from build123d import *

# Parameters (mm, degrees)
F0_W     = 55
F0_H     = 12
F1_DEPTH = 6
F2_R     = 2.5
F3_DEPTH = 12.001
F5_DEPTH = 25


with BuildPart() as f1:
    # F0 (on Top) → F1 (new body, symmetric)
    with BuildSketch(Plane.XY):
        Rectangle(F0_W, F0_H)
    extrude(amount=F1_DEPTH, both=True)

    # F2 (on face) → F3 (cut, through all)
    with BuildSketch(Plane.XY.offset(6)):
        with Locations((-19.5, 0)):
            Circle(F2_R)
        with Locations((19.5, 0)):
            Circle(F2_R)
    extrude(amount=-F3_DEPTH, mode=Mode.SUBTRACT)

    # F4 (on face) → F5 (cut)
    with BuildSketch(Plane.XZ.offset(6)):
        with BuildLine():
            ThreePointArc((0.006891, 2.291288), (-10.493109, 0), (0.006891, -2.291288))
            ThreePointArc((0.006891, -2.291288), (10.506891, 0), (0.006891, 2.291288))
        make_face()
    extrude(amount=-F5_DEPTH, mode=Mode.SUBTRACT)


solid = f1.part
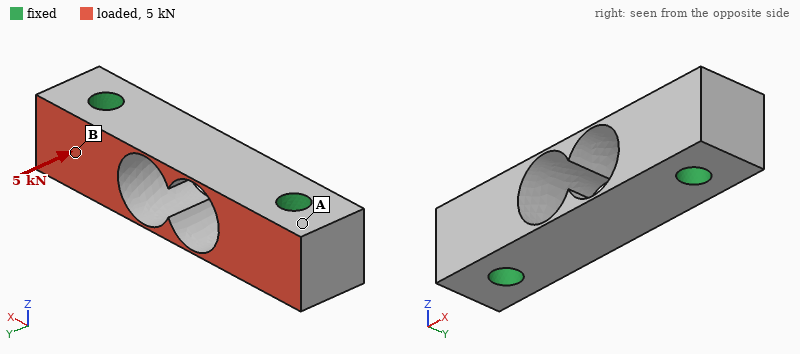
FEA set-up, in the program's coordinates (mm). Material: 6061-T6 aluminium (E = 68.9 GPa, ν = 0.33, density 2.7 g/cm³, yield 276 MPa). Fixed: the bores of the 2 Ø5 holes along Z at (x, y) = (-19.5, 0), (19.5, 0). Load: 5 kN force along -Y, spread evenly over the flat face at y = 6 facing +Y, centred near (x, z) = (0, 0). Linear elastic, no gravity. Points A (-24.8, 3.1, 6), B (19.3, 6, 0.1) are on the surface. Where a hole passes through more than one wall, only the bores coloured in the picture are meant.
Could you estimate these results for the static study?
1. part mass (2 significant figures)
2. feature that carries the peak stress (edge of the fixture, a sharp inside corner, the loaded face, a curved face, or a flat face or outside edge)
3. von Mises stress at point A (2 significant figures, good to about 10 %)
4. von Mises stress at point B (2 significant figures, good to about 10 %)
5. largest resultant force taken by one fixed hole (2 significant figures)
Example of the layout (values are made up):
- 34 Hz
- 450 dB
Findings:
- 14 g
- the loaded face
- 9.5 MPa
- 29 MPa
- 2.5 kN
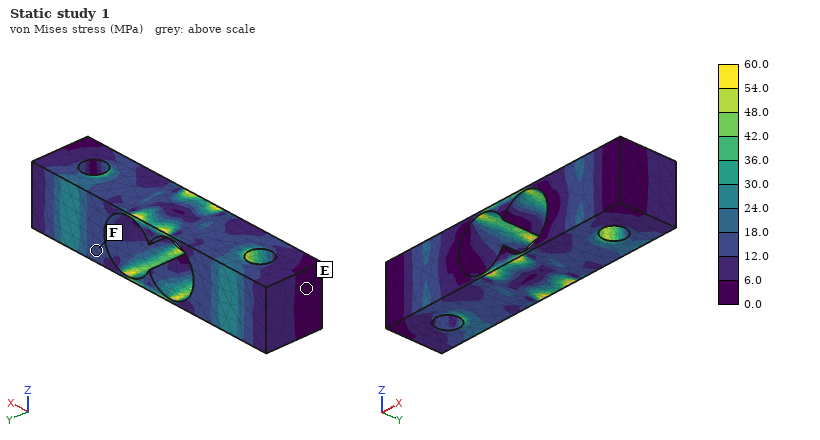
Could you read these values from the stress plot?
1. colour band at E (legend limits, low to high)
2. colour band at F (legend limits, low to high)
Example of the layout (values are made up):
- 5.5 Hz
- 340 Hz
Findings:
- 0.0 to 6.0 MPa
- 12.0 to 18.0 MPa
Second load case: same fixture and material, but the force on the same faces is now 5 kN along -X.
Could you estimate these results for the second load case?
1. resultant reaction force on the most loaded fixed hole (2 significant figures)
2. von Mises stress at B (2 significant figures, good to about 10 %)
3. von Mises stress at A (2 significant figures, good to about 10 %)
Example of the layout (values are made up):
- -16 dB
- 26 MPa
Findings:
- 2.5 kN
- 18 MPa
- 10 MPa
